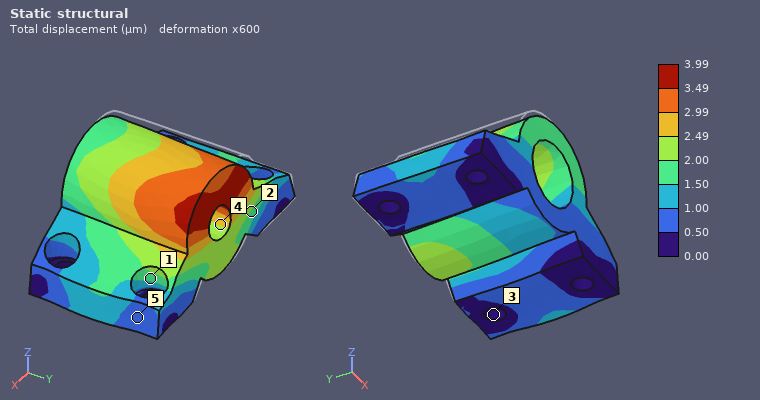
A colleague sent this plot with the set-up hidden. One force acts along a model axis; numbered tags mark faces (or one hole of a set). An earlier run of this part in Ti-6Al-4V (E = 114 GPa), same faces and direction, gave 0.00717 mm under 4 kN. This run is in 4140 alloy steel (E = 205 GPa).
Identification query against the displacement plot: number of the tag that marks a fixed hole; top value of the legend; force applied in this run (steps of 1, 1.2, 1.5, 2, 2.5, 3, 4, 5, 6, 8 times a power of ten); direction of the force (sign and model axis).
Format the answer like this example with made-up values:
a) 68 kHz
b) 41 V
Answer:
a) 3
b) 3.99 µm
c) 4 kN
d) +X
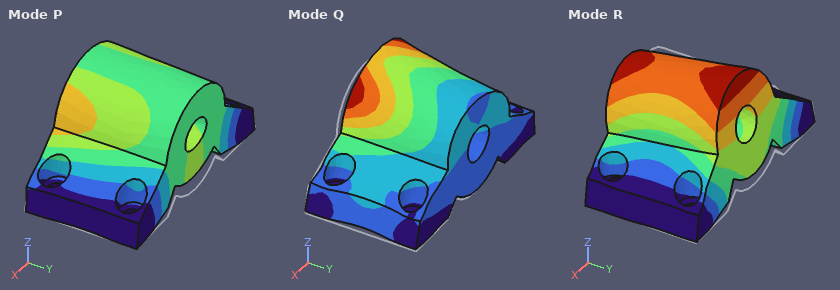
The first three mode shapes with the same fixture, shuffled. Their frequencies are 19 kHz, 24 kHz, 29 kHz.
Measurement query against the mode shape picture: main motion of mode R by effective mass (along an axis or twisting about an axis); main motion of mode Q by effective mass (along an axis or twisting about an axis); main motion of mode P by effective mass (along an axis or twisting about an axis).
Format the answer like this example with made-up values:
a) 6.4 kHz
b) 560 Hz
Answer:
a) along Y
b) along X
c) along Z
